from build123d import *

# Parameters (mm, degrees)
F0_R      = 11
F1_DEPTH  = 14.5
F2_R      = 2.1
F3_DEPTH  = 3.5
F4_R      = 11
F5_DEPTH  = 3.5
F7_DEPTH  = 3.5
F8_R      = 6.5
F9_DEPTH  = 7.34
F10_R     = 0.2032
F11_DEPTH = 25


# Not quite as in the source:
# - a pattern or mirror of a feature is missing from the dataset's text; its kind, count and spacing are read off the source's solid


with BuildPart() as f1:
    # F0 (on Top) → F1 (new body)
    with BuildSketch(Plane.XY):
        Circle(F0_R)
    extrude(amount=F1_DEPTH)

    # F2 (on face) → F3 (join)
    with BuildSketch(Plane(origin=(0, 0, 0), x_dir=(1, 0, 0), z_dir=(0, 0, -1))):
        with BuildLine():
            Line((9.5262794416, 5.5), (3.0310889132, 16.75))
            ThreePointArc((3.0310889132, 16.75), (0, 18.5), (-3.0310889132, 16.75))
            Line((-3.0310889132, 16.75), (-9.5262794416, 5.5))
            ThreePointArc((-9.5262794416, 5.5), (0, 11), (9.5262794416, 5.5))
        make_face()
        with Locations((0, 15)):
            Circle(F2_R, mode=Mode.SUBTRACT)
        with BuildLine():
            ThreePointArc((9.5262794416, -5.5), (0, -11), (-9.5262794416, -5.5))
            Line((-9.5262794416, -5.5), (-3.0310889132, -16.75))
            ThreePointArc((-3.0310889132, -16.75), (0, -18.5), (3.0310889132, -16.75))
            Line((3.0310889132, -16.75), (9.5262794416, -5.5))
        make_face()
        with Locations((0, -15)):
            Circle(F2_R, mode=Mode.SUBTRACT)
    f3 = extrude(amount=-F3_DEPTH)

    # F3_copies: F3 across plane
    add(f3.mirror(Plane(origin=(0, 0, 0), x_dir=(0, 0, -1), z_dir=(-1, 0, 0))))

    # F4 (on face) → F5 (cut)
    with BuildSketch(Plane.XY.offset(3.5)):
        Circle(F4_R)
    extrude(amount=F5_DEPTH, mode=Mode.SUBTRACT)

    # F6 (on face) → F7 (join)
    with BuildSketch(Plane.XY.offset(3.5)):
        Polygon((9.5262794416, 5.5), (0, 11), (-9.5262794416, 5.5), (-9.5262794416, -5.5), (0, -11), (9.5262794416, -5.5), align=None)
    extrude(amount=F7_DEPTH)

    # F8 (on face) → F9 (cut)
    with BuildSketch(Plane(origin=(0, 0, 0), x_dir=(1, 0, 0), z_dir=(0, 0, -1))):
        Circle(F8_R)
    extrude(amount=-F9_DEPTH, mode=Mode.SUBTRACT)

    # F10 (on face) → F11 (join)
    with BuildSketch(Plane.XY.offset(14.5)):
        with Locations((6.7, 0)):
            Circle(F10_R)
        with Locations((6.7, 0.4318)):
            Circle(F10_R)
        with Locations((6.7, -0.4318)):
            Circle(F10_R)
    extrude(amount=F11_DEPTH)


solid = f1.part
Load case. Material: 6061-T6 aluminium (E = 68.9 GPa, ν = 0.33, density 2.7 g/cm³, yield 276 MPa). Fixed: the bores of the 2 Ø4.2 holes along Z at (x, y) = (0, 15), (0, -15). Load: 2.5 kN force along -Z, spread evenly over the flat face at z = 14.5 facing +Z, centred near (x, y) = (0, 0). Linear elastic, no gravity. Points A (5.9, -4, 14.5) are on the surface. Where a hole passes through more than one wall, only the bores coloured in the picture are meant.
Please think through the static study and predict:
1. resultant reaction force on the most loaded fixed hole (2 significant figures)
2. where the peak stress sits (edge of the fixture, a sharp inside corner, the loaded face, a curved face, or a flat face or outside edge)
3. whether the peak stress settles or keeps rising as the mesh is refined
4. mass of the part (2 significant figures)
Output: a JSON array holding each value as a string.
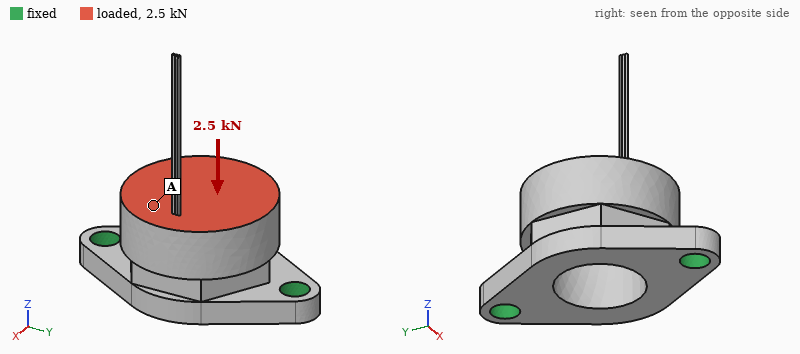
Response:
["1.4 kN", "edge of the fixture", "keeps rising", "13 g"]
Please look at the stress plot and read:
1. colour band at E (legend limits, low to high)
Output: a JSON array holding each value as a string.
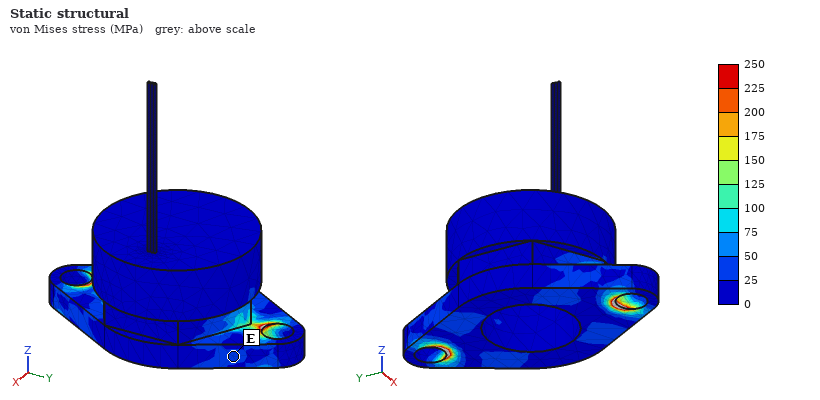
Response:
["25 to 50 MPa"]
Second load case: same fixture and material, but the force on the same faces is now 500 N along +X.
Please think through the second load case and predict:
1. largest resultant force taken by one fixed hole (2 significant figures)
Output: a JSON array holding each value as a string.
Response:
["250 N"]
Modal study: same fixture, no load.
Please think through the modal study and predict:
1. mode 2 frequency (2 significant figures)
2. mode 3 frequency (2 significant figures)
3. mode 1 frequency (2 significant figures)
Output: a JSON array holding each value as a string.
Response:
["460 Hz", "460 Hz", "460 Hz"]
